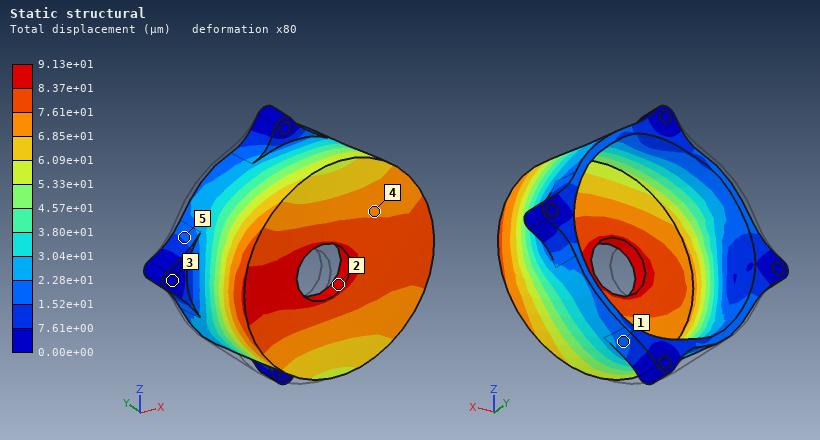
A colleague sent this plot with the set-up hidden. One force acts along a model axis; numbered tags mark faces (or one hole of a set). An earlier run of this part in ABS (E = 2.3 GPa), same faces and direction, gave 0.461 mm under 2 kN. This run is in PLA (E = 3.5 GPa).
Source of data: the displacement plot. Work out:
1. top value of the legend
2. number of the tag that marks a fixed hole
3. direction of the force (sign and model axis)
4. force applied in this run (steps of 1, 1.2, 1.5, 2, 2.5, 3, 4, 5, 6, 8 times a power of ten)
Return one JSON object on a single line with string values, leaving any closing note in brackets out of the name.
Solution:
{"top value of the legend": "9.13e+01 µm", "number of the tag that marks a fixed hole": "3", "direction of the force": "+X", "force applied in this run": "600 N"}
